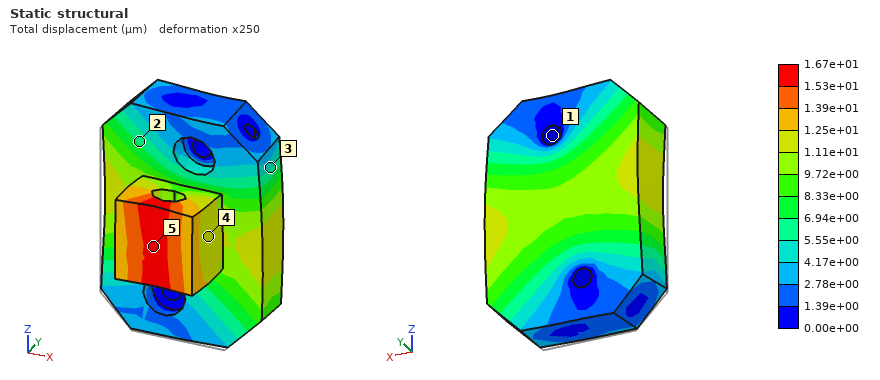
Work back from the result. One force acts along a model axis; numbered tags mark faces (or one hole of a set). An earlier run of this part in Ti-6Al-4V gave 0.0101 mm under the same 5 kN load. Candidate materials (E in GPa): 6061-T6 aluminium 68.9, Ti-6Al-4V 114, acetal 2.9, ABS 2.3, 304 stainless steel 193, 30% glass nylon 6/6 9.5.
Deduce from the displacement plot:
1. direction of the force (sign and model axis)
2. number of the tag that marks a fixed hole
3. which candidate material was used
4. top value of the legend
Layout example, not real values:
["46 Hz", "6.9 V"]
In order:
["+Y", "1", "6061-T6 aluminium", "1.67e+01 µm"]
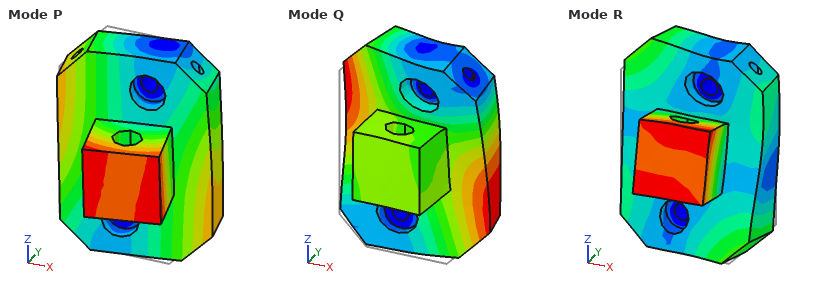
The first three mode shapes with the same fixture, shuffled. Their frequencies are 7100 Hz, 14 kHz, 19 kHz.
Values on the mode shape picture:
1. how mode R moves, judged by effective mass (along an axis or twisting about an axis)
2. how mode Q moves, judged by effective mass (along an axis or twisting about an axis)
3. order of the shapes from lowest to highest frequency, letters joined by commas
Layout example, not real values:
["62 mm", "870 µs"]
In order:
["along Z", "along Y", "P, Q, R"]
